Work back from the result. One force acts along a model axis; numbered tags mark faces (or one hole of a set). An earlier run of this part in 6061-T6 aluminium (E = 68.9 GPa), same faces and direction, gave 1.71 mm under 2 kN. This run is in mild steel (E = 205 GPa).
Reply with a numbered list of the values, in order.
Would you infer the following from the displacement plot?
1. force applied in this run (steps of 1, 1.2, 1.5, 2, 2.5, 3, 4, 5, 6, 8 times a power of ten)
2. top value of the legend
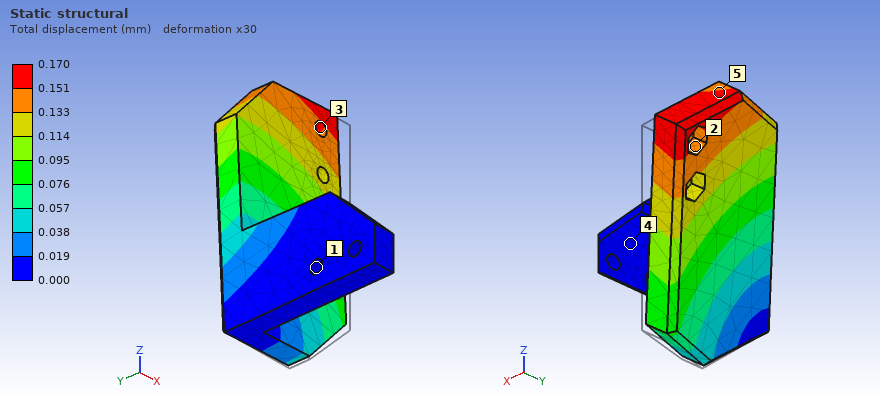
1. 600 N
2. 0.170 mm
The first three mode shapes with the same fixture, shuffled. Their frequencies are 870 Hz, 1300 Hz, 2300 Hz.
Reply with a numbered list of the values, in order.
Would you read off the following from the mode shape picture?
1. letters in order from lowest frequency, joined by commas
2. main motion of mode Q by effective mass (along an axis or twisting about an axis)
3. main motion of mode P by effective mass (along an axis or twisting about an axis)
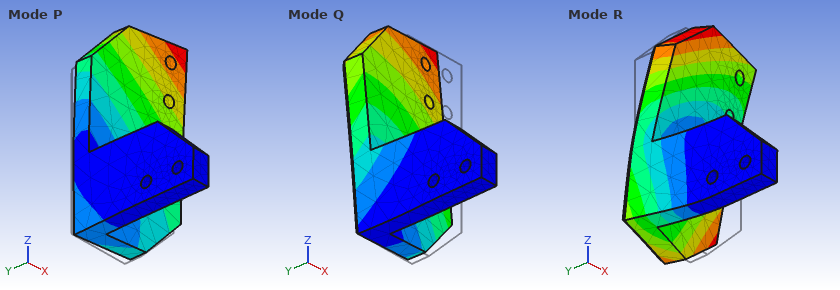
1. Q, P, R
2. along X
3. along Y
